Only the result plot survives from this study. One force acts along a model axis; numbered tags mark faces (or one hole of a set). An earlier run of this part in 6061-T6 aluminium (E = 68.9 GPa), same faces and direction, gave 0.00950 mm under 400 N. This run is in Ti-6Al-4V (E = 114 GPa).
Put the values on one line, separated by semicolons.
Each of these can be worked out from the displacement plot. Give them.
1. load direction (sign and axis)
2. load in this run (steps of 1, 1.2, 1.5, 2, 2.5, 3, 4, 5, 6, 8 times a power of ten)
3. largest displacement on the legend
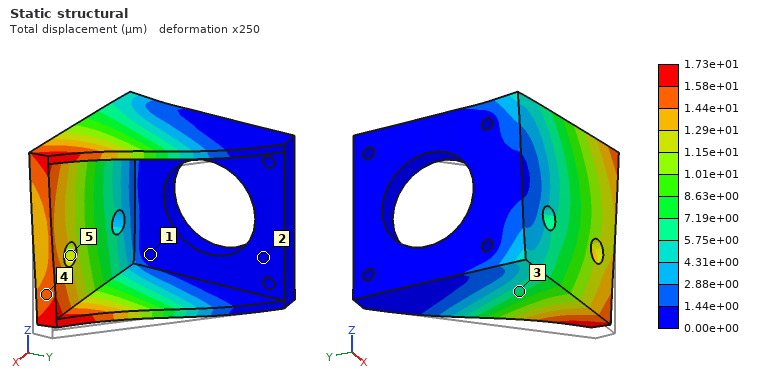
+Z; 1.2 kN; 1.73e+01 µm
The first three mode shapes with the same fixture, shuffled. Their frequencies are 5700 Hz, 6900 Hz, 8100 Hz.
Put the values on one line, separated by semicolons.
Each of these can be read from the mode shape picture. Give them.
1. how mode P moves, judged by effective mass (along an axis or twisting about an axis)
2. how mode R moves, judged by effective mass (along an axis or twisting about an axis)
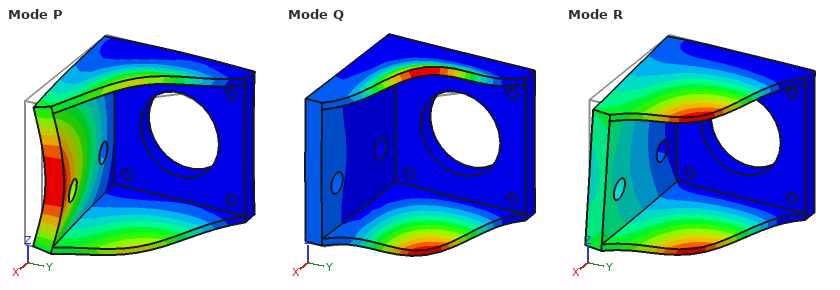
along Y; along Z
